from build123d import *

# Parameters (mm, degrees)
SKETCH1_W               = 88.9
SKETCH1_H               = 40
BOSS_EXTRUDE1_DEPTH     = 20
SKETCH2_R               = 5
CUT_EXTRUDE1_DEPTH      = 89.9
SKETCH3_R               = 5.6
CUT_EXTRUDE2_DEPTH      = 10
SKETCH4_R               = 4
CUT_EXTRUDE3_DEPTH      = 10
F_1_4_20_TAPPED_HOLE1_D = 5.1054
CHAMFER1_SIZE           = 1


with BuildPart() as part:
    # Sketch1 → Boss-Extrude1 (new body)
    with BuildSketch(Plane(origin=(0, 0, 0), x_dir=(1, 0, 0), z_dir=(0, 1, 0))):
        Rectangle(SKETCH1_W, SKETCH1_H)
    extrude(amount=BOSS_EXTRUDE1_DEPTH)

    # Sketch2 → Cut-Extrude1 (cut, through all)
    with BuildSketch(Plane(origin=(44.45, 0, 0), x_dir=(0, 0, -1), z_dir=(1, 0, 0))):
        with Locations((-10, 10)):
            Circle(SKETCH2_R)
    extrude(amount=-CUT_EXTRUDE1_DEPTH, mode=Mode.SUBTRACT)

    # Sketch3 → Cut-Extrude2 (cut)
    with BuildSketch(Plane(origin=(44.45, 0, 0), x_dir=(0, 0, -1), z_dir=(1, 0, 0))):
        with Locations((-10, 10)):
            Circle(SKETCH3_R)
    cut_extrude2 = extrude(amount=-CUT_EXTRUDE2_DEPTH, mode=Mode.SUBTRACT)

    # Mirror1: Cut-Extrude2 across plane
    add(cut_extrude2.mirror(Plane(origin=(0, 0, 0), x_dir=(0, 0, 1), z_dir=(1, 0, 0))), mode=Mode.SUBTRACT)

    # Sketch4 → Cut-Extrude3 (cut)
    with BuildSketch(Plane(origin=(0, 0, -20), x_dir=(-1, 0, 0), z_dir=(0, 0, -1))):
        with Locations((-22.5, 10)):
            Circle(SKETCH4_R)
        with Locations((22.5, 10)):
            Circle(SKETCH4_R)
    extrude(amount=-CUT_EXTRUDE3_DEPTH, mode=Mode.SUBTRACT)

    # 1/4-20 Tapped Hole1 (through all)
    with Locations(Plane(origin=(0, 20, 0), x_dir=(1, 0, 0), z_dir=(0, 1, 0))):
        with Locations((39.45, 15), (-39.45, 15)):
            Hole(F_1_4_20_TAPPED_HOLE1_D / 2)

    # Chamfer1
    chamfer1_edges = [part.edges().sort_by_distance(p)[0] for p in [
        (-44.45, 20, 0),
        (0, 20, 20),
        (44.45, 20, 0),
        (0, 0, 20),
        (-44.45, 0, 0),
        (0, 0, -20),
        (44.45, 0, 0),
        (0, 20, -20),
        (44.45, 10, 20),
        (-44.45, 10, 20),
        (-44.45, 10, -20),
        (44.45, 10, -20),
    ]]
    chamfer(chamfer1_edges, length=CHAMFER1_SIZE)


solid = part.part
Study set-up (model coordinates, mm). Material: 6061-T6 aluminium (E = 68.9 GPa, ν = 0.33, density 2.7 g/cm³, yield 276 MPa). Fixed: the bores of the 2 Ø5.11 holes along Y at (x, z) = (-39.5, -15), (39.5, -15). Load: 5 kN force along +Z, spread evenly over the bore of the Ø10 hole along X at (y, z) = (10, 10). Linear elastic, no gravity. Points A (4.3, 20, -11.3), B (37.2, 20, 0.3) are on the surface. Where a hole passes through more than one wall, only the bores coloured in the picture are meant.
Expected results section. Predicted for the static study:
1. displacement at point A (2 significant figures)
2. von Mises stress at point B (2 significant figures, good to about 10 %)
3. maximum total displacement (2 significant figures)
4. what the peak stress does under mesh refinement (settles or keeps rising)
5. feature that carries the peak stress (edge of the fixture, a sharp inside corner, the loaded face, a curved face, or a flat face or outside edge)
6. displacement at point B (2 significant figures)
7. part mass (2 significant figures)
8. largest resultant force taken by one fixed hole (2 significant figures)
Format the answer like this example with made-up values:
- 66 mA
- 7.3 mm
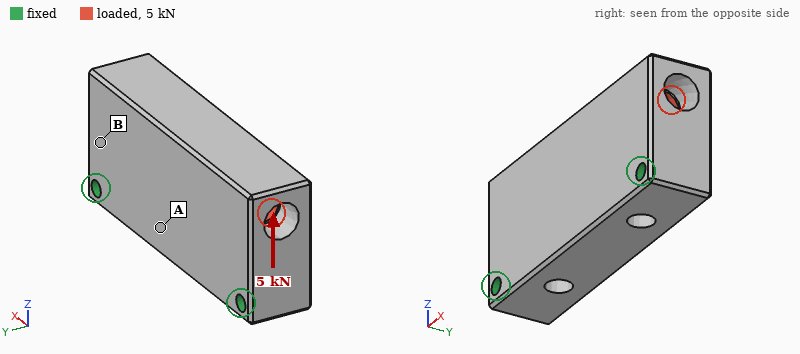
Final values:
- 6.9 µm
- 6.5 MPa
- 7.9 µm
- keeps rising
- edge of the fixture
- 1.9 µm
- 170 g
- 2.9 kN
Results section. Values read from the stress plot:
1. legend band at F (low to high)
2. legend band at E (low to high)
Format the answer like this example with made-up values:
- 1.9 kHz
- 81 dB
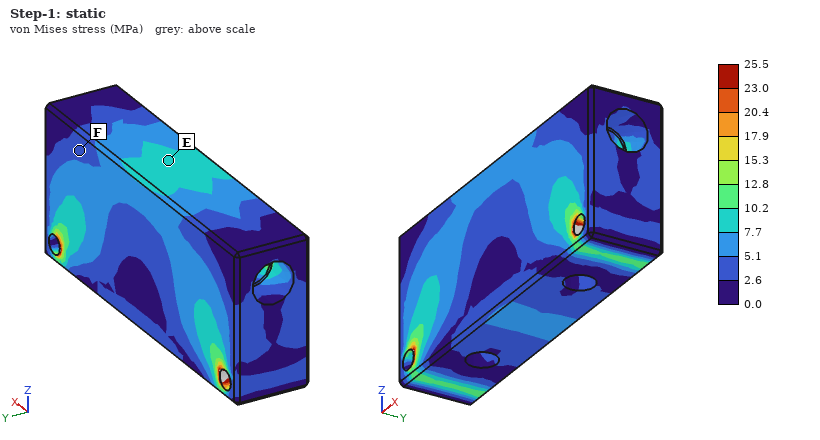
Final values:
- 2.6 to 5.1 MPa
- 7.7 to 10.2 MPa
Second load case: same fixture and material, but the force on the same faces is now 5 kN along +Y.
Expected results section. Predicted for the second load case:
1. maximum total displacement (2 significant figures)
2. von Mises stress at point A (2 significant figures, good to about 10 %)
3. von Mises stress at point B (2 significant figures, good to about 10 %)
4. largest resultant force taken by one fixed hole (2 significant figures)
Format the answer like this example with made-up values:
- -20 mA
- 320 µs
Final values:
- 56 µm
- 9.7 MPa
- 23 MPa
- 2.5 kN
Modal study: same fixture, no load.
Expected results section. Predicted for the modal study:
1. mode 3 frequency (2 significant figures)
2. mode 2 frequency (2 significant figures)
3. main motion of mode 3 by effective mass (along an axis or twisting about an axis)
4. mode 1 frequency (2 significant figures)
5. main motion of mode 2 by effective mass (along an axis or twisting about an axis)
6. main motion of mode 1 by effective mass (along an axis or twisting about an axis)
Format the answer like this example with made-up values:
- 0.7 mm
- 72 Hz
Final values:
- 12 kHz
- 12 kHz
- twisting about Z
- 6300 Hz
- along Y
- along Y
